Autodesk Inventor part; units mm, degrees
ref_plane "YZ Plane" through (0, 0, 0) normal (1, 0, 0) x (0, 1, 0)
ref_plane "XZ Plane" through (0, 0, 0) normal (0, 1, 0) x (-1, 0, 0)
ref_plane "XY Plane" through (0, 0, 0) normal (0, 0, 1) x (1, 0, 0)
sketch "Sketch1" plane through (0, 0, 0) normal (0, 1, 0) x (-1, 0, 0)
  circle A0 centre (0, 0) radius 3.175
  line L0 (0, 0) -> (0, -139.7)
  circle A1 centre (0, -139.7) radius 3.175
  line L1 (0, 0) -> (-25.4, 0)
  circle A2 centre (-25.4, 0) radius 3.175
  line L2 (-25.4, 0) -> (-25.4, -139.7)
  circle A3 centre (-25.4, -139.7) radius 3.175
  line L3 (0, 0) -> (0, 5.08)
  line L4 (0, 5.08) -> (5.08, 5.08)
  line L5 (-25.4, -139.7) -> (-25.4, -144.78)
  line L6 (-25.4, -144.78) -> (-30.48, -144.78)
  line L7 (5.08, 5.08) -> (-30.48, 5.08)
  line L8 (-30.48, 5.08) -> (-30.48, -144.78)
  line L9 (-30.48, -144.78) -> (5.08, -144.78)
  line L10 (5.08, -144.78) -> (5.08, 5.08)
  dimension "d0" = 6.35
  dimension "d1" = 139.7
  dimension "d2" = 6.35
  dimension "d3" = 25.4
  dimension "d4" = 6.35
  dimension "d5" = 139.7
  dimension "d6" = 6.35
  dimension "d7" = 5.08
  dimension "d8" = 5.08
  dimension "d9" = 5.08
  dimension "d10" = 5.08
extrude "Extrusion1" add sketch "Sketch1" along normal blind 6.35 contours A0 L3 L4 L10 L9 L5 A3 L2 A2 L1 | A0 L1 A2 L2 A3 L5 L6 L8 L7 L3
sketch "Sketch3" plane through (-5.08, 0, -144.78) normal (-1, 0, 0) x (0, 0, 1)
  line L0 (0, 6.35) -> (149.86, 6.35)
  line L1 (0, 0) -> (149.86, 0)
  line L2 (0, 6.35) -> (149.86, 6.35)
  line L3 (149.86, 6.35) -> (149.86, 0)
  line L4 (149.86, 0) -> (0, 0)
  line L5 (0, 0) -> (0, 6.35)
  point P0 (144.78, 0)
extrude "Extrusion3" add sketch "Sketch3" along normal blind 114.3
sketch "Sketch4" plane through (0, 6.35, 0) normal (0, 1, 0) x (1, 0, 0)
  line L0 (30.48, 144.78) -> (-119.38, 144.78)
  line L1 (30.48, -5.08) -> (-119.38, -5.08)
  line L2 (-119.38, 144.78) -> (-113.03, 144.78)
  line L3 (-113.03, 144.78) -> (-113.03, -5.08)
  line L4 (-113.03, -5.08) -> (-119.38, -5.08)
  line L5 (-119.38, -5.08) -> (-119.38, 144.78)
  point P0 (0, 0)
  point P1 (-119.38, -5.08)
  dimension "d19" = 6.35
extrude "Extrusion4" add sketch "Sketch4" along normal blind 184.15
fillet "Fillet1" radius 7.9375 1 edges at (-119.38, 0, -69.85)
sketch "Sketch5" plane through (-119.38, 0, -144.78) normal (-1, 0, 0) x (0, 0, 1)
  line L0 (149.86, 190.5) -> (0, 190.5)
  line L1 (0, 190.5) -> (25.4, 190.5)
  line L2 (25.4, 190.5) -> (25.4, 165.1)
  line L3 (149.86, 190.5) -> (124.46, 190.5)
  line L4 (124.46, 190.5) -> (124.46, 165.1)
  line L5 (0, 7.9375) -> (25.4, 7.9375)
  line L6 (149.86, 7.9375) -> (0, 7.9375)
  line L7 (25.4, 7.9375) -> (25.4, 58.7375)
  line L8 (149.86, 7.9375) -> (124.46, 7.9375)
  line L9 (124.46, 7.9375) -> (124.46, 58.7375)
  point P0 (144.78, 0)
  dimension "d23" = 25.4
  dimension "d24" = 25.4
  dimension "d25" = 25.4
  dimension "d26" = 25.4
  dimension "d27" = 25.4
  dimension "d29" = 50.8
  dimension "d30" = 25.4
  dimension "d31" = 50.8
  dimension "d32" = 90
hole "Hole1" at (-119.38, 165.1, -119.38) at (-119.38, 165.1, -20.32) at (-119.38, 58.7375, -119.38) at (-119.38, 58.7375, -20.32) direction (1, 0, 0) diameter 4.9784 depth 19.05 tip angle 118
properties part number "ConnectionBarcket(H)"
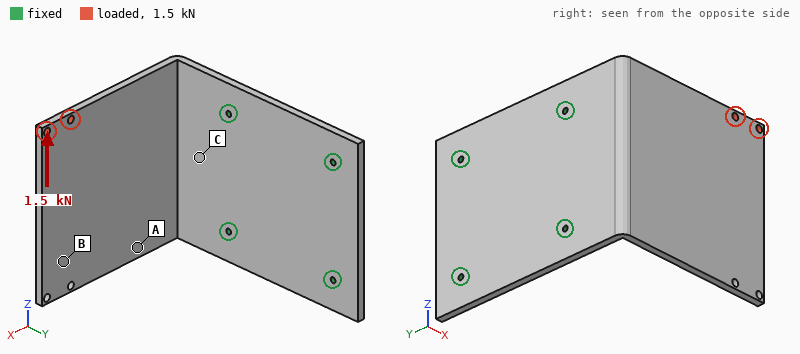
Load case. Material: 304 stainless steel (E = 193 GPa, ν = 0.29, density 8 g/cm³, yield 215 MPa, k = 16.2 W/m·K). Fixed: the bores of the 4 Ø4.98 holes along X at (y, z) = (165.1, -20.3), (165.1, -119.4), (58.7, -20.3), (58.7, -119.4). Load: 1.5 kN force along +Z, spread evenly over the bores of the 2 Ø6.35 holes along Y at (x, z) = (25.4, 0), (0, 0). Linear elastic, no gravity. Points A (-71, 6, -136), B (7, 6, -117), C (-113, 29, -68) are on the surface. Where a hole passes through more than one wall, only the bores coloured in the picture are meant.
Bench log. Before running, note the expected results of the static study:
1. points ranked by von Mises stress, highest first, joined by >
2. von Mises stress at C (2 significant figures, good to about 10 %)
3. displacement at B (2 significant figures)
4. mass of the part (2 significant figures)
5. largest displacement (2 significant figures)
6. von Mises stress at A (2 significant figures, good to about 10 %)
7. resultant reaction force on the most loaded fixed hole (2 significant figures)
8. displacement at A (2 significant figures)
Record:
C > A > B
71 MPa
0.56 mm
2.5 kg
0.71 mm
33 MPa
2.2 kN
0.35 mm
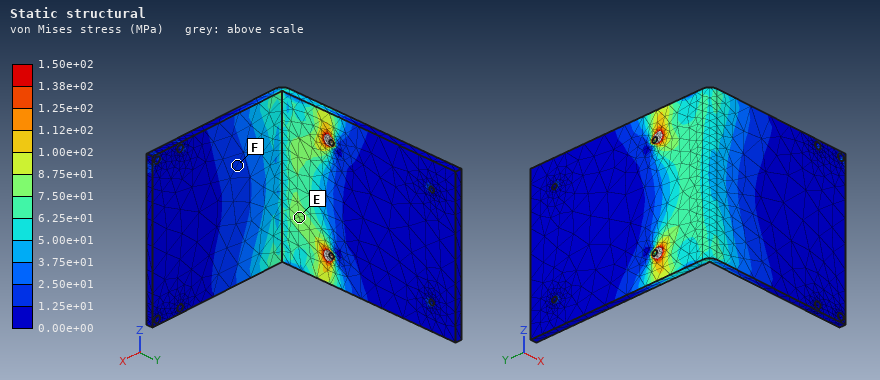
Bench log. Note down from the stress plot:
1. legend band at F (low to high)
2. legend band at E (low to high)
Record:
1.25e+01 to 2.50e+01 MPa
7.50e+01 to 8.75e+01 MPa
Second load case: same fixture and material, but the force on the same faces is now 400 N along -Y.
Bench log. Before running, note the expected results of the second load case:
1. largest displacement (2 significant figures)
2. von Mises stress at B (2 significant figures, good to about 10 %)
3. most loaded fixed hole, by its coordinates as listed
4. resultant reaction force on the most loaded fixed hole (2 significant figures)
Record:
1.5 mm
12 MPa
(58.7, -20.3)
380 N
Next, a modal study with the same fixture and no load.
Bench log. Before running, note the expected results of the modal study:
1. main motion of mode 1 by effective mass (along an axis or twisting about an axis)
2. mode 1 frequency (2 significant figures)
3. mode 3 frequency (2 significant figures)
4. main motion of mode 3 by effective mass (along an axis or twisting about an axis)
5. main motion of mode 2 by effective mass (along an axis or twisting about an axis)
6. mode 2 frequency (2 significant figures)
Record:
along Y
140 Hz
560 Hz
along X
along Z
330 Hz
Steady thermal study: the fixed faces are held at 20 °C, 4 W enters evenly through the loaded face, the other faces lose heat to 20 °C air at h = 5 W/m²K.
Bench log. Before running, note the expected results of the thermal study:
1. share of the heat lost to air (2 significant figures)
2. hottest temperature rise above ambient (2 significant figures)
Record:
80 %
57 K
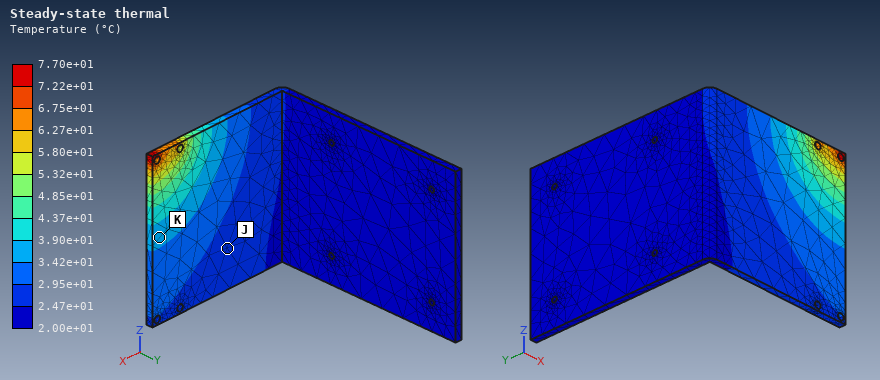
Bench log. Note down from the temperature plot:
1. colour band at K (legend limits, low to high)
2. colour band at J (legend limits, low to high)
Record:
3.42e+01 to 3.90e+01 °C
2.47e+01 to 2.95e+01 °C
